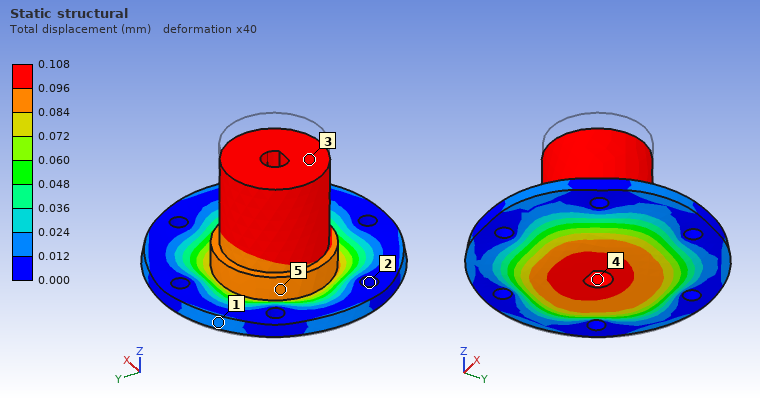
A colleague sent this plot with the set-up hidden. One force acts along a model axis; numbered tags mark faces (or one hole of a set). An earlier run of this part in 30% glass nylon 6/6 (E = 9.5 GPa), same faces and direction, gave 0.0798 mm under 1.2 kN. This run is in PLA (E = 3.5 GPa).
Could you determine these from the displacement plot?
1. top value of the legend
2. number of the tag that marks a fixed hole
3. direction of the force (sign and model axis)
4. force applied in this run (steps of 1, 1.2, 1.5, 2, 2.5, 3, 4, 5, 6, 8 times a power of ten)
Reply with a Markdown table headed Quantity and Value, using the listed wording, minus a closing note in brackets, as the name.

| Quantity | Value |
|---|---|
| top value of the legend | 0.108 mm |
| number of the tag that marks a fixed hole | 2 |
| direction of the force | -Z |
| force applied in this run | 600 N |
